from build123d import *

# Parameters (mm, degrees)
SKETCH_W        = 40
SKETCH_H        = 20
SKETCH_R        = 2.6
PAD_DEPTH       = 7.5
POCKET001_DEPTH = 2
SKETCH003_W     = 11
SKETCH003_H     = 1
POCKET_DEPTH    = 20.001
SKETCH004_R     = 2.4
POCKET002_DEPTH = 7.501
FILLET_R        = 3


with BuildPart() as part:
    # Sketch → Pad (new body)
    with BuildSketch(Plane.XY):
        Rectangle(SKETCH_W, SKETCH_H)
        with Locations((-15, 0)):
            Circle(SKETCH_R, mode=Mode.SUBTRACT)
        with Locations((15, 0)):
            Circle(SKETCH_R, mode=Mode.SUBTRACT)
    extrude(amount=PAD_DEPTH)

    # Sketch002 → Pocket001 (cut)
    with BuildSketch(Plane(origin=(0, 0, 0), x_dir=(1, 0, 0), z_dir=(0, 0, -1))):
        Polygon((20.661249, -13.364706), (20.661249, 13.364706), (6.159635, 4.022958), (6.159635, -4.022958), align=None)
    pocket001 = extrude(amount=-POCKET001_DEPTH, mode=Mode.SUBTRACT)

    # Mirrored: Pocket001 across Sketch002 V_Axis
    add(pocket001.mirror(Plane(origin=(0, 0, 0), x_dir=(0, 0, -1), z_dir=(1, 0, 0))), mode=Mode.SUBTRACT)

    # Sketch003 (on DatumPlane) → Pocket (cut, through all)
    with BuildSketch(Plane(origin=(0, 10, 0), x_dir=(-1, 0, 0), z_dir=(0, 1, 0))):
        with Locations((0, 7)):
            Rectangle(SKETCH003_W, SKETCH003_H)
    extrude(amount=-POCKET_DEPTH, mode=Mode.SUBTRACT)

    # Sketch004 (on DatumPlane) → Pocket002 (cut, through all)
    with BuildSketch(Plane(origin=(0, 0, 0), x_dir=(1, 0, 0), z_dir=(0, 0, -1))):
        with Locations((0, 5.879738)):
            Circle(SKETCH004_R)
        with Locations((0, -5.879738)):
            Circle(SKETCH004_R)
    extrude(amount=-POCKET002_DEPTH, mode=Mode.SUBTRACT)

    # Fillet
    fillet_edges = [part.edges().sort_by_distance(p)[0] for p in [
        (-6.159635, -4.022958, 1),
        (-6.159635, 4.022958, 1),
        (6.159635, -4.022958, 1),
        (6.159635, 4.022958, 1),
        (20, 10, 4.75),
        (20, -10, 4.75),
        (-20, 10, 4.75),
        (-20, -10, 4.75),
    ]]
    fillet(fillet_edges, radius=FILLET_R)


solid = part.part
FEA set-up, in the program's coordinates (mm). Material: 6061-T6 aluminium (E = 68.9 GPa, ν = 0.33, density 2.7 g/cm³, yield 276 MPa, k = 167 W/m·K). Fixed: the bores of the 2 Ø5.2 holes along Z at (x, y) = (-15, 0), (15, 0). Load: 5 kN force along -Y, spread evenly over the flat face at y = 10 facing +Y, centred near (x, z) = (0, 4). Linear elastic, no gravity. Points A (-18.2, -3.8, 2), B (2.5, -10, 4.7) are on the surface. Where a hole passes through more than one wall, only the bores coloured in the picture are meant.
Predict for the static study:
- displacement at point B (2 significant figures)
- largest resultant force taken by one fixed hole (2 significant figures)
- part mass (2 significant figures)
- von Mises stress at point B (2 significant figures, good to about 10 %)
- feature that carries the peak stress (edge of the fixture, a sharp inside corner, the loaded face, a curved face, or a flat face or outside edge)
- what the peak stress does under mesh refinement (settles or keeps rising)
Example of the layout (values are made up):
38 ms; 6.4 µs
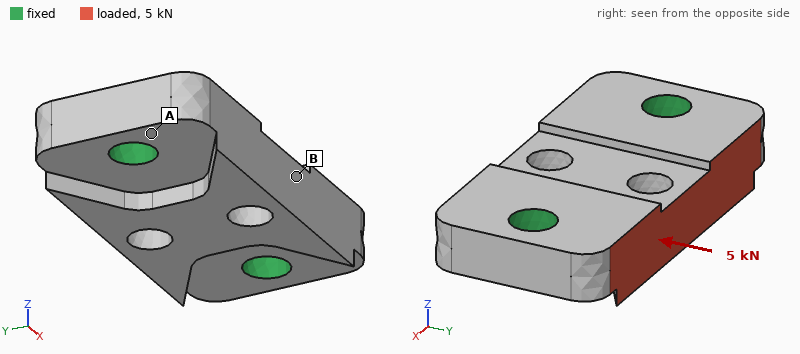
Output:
10 µm; 2.5 kN; 12 g; 45 MPa; edge of the fixture; keeps rising
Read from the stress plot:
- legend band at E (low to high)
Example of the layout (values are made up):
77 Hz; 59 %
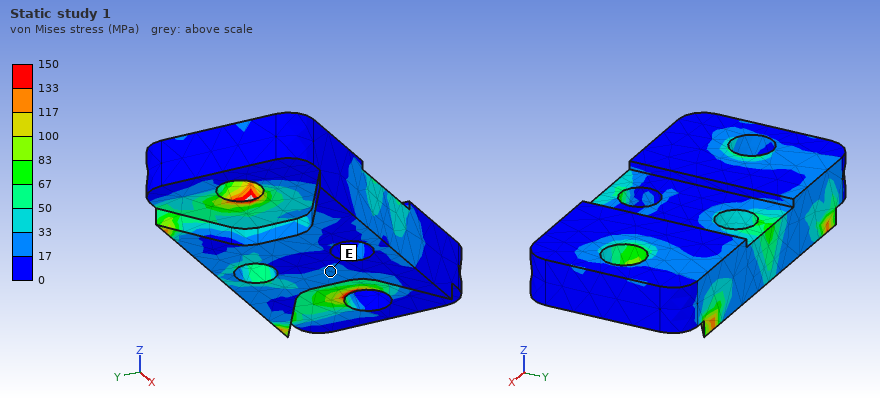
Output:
17 to 33 MPa
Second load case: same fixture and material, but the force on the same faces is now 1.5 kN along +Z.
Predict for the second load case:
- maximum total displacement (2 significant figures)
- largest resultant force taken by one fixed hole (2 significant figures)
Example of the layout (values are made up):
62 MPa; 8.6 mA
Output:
33 µm; 790 N
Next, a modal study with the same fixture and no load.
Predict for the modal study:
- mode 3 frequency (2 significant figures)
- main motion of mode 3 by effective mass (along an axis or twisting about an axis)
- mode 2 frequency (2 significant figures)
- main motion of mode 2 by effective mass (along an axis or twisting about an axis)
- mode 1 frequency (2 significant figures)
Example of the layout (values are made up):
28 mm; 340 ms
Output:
39 kHz; along Y; 27 kHz; along Z; 25 kHz
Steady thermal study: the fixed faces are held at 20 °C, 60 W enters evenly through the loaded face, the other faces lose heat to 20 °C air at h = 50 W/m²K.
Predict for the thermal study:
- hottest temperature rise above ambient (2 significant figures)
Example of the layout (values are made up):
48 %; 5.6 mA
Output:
26 K
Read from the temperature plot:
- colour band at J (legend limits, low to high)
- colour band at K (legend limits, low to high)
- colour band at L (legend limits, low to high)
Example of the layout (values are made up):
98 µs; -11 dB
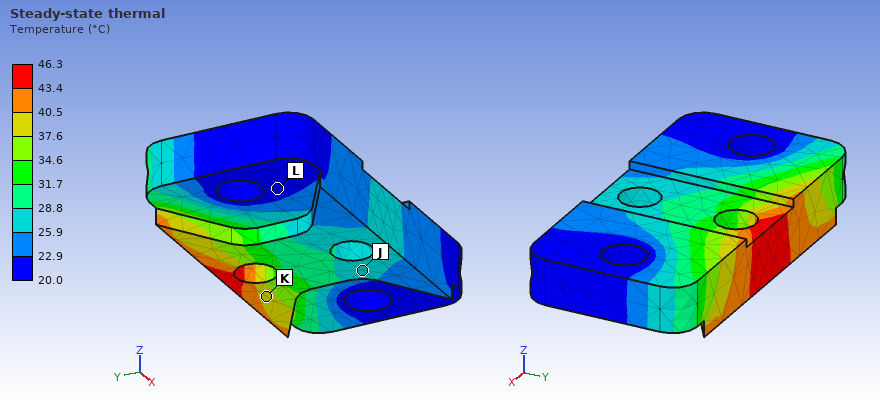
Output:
25.9 to 28.8 °C; 37.6 to 40.5 °C; 20.0 to 22.9 °C
